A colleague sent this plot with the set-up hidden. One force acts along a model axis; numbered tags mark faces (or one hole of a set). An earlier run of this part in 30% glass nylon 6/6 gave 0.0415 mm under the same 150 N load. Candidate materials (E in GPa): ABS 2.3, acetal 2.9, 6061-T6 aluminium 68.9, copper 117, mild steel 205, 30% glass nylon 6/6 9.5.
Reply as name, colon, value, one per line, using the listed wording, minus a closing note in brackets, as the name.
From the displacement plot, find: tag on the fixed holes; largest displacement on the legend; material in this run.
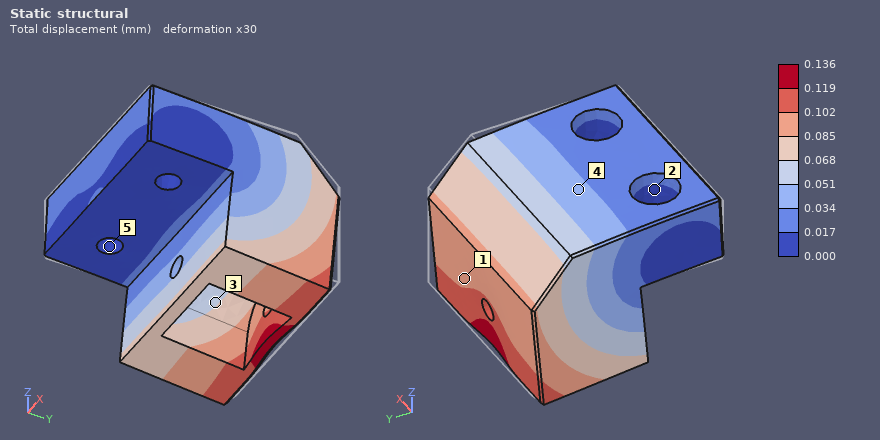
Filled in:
tag on the fixed holes: 5
largest displacement on the legend: 0.136 mm
material in this run: acetal
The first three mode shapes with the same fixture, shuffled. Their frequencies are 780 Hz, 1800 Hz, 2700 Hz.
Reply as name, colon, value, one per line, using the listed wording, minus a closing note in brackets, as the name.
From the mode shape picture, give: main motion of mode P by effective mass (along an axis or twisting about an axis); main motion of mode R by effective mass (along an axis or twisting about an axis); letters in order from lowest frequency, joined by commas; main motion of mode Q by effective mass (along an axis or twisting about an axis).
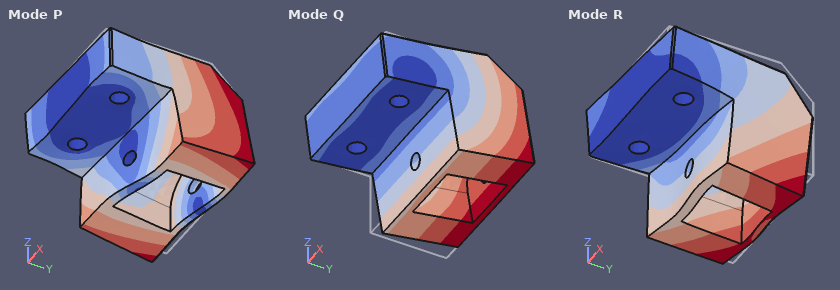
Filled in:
main motion of mode P by effective mass: along X
main motion of mode R by effective mass: along X
letters in order from lowest frequency, joined by commas: Q, R, P
main motion of mode Q by effective mass: along Z
